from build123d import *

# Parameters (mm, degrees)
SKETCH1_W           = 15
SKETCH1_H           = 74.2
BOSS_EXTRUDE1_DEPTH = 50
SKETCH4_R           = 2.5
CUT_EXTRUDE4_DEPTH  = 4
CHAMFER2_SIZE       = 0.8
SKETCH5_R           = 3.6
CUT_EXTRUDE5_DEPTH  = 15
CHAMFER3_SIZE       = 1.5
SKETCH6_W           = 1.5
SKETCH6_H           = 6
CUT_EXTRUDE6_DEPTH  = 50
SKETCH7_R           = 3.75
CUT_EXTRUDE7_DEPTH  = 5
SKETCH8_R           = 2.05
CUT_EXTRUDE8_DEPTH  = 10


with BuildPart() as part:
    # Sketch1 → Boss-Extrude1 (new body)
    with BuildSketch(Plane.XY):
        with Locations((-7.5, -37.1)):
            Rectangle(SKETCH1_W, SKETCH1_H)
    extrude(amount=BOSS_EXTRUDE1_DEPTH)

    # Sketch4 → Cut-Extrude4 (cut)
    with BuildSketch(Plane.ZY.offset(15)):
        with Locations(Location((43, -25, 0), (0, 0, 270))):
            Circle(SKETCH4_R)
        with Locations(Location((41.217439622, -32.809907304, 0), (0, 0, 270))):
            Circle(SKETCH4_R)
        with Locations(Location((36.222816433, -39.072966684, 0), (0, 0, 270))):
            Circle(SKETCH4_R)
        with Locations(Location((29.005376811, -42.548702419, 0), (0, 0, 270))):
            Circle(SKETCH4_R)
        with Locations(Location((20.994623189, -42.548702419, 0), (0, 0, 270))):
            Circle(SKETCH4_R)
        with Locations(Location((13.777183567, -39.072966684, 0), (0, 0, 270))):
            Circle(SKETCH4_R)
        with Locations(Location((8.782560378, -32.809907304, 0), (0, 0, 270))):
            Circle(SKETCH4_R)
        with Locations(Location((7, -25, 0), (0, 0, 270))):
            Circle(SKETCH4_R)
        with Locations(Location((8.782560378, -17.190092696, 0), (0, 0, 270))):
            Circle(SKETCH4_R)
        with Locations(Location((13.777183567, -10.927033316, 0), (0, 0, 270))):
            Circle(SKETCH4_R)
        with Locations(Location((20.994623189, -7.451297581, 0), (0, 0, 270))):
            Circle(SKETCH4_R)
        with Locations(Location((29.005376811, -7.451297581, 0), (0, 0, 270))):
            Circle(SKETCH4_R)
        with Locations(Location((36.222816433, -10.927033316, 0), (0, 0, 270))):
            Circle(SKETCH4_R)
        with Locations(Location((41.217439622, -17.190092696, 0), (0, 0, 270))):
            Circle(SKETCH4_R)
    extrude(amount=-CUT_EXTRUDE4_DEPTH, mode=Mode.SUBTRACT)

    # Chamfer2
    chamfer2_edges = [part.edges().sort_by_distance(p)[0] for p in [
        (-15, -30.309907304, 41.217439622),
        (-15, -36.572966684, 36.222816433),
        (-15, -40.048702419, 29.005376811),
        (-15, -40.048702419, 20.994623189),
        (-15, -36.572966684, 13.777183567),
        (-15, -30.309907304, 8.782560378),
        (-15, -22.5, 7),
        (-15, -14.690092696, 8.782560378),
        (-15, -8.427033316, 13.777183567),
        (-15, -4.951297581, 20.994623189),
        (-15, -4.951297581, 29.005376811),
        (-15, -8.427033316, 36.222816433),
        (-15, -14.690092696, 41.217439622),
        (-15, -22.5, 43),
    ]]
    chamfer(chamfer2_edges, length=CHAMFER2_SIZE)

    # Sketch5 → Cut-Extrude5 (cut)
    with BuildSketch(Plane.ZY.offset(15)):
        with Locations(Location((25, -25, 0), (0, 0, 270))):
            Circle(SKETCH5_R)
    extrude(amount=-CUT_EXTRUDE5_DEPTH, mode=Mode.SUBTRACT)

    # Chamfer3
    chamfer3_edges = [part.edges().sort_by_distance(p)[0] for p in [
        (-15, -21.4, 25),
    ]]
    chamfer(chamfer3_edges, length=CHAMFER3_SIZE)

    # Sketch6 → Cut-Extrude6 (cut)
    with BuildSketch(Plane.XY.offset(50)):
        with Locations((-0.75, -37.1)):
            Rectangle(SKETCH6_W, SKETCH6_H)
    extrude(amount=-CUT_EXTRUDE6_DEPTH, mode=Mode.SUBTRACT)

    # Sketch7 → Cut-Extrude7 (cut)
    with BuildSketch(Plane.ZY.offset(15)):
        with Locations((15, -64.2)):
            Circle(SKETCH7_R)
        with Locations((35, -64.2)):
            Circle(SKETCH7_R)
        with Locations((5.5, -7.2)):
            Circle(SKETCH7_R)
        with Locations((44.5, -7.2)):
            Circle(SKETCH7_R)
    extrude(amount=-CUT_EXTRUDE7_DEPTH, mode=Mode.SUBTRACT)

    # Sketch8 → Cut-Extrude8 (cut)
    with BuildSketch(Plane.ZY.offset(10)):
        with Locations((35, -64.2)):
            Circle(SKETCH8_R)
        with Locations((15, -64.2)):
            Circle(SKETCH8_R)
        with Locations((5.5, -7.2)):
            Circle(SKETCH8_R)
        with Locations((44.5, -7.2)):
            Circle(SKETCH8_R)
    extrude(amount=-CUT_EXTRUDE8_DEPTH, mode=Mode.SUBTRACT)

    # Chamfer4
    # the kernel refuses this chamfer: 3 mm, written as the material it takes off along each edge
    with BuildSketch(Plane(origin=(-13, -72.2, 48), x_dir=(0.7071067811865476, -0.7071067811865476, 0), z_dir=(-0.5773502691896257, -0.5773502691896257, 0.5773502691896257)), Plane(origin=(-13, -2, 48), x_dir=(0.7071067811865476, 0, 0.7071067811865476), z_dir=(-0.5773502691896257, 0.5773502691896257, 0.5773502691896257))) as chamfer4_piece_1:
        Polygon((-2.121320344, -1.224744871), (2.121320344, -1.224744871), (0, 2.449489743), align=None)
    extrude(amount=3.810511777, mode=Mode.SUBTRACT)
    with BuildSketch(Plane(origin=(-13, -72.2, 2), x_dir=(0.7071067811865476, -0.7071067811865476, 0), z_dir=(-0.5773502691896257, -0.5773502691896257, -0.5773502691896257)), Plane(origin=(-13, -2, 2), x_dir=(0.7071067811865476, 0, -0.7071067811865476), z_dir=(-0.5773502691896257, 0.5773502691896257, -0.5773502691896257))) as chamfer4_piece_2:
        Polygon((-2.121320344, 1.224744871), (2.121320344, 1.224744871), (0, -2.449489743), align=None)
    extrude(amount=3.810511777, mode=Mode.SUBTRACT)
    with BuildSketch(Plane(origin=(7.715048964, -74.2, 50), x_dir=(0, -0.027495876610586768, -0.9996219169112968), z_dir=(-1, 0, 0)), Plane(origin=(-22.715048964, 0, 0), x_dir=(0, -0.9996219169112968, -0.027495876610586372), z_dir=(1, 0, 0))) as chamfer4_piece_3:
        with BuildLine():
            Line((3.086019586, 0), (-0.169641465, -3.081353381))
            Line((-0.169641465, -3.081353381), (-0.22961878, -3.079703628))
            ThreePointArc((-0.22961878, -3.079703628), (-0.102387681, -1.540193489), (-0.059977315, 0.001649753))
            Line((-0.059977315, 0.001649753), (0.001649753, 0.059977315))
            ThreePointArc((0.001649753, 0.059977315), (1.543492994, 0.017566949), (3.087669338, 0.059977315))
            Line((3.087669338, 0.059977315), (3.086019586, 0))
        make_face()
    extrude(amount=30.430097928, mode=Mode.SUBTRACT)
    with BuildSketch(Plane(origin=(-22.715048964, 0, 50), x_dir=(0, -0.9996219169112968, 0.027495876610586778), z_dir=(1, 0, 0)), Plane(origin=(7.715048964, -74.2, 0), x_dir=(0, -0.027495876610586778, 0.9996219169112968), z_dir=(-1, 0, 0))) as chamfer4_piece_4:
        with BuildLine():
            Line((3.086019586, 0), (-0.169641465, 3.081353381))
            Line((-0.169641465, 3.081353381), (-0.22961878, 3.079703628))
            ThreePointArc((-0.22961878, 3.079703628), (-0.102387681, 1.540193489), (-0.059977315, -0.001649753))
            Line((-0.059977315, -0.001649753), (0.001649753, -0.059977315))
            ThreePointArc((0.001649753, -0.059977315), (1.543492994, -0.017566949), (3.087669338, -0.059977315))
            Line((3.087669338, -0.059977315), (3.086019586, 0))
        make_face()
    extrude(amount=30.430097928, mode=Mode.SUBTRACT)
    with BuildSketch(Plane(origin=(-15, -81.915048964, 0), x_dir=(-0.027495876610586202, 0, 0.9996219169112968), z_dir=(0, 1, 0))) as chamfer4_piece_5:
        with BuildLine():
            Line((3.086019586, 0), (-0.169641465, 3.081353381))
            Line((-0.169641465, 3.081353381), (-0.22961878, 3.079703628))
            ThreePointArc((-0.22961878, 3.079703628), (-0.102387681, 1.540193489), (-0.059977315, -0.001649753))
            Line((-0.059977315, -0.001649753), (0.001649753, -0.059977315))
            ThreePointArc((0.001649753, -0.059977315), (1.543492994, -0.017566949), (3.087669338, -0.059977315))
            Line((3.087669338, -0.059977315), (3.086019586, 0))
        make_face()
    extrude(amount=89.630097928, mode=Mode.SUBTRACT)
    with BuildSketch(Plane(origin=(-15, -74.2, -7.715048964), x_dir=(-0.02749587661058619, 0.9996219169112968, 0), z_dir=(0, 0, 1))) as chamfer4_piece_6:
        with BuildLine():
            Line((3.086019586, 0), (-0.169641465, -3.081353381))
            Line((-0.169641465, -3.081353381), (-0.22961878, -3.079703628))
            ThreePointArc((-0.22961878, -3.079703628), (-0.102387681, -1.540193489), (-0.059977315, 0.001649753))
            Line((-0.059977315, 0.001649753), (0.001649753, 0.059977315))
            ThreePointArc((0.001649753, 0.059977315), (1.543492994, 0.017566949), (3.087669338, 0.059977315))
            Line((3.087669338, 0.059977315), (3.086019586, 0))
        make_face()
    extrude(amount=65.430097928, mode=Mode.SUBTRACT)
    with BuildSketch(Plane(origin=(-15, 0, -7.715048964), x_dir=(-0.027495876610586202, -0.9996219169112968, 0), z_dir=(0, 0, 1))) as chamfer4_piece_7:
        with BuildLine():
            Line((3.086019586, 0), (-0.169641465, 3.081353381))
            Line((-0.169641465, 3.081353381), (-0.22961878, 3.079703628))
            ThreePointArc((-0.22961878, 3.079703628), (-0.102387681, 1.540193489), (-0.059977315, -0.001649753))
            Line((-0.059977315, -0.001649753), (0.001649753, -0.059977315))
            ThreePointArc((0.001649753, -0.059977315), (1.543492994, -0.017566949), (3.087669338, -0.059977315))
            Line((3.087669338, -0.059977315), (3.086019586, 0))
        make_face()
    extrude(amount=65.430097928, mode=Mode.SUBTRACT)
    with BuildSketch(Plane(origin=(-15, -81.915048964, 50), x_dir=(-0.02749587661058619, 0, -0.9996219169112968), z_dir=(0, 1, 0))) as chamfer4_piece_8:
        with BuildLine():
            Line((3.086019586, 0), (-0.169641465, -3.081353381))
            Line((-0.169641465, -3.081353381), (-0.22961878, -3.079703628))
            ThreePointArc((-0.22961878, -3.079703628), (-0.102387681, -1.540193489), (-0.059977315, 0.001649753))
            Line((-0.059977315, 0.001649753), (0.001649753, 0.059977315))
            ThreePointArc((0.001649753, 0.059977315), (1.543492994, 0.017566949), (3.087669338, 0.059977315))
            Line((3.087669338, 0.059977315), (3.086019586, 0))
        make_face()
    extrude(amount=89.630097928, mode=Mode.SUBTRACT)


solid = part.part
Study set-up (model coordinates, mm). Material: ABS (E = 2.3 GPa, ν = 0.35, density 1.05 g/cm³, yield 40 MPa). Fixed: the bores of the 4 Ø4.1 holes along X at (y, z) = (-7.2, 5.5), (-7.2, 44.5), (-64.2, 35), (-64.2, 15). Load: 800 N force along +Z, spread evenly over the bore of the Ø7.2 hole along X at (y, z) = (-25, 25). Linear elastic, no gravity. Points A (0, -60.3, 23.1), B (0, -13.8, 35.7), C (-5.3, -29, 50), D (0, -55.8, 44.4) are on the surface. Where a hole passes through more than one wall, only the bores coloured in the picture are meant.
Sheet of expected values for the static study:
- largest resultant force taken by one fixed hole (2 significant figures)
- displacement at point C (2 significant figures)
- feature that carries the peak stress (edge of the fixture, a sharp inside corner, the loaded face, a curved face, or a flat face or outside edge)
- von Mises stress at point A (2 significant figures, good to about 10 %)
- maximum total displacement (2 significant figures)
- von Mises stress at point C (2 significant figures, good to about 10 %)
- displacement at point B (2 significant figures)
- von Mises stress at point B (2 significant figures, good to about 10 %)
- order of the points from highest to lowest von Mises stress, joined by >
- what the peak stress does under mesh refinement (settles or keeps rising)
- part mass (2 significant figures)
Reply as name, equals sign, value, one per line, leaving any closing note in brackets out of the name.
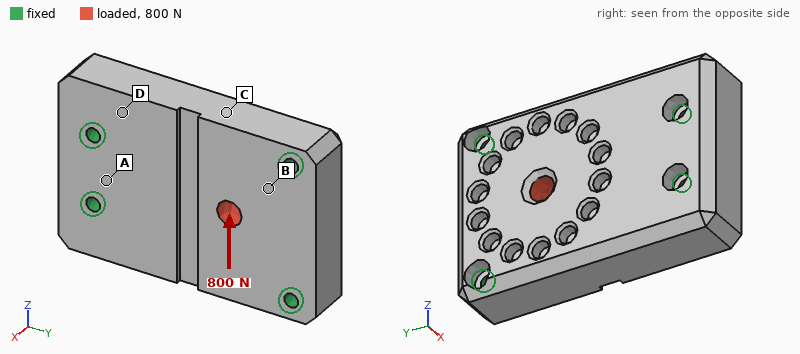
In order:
largest resultant force taken by one fixed hole = 310 N
displacement at point C = 21 µm
feature that carries the peak stress = edge of the fixture
von Mises stress at point A = 0.91 MPa
maximum total displacement = 32 µm
von Mises stress at point C = 1.5 MPa
displacement at point B = 12 µm
von Mises stress at point B = 2.2 MPa
order of the points from highest to lowest von Mises stress, joined by > = B > C > A > D
what the peak stress does under mesh refinement = keeps rising
part mass = 53 g
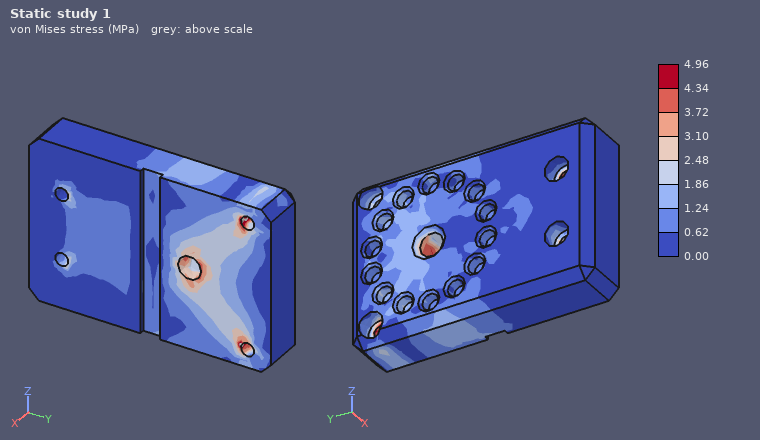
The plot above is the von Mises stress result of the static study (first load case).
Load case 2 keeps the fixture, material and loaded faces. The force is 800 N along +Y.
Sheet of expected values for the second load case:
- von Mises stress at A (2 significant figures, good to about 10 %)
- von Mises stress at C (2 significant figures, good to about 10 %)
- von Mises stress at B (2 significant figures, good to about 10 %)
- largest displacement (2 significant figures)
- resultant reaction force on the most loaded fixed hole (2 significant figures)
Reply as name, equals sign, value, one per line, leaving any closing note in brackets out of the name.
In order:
von Mises stress at A = 0.45 MPa
von Mises stress at C = 0.37 MPa
von Mises stress at B = 1.5 MPa
largest displacement = 24 µm
resultant reaction force on the most loaded fixed hole = 240 N
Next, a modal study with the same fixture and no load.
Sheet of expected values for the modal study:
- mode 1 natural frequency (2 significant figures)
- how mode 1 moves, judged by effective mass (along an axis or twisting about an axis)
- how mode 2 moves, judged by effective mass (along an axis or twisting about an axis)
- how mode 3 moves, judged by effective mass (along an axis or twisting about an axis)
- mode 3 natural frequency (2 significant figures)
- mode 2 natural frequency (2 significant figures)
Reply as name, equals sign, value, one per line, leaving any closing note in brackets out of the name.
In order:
mode 1 natural frequency = 3500 Hz
how mode 1 moves, judged by effective mass = along X
how mode 2 moves, judged by effective mass = twisting about Y
how mode 3 moves, judged by effective mass = along Z
mode 3 natural frequency = 5800 Hz
mode 2 natural frequency = 4500 Hz
